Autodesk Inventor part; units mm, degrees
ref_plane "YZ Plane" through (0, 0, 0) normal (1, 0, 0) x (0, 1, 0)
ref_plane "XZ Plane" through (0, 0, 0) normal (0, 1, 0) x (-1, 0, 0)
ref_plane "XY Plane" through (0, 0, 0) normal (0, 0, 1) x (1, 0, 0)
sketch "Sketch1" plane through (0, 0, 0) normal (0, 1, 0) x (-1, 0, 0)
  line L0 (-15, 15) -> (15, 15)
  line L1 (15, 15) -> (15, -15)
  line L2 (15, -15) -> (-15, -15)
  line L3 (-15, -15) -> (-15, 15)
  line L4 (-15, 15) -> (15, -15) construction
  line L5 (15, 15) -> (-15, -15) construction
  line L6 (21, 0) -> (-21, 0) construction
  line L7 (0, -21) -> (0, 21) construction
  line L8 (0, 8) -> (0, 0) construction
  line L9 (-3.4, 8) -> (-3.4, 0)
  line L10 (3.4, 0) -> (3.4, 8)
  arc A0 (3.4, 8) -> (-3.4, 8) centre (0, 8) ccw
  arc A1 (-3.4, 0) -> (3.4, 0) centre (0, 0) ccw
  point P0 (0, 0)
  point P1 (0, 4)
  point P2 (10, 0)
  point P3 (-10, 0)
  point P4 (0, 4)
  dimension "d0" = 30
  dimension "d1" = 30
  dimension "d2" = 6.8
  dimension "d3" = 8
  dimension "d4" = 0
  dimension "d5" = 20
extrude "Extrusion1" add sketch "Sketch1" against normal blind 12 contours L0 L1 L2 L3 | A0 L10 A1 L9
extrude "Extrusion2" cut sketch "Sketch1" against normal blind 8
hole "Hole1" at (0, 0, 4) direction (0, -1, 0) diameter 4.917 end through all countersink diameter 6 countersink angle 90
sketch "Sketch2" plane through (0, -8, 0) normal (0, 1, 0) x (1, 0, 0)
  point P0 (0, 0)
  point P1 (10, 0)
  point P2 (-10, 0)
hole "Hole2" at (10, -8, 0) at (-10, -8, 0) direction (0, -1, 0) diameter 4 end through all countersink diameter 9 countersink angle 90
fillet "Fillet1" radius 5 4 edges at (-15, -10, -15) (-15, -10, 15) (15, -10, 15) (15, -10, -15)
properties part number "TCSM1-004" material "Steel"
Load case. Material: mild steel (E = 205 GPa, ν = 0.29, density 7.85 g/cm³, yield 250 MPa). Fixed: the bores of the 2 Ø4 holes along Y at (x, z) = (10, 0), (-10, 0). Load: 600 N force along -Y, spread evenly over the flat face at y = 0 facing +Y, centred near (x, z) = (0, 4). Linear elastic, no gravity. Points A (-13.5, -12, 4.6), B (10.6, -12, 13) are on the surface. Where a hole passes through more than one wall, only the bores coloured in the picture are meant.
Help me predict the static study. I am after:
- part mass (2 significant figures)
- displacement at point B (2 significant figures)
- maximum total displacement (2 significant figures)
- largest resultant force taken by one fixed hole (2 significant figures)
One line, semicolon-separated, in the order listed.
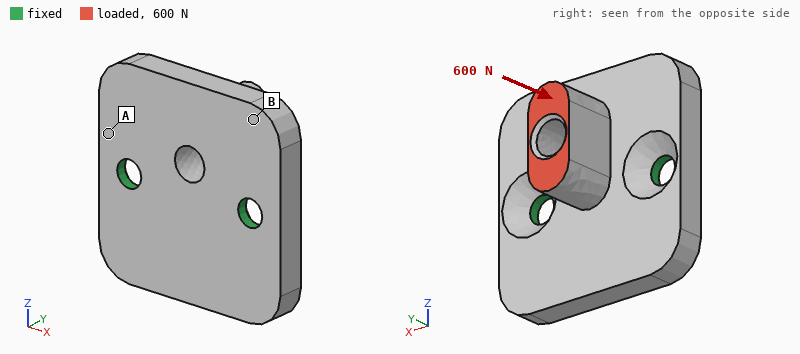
30 g; 8.3 µm; 12 µm; 380 N
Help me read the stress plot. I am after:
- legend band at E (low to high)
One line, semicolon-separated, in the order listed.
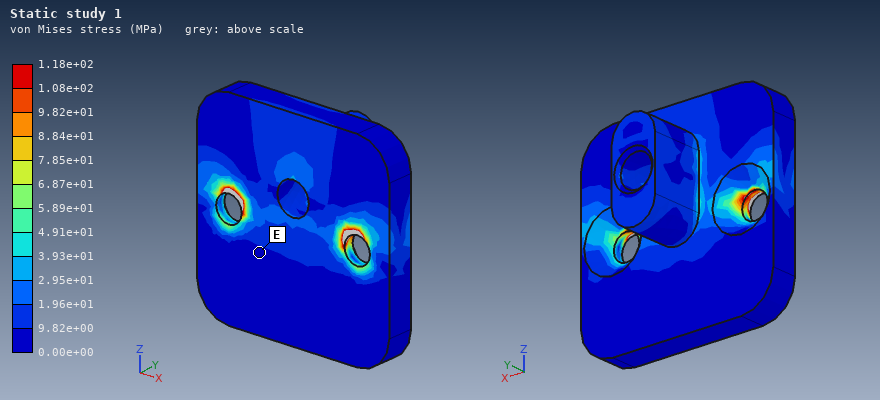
0.00e+00 to 9.82e+00 MPa
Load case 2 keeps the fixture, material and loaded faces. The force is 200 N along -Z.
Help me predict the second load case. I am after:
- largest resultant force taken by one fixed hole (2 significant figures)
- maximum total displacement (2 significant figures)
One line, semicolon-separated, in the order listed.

100 N; 9.9 µm
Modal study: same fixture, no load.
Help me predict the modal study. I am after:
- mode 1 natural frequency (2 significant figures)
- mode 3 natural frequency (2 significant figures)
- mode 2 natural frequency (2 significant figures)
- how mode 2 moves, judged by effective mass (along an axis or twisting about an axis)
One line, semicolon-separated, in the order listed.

7000 Hz; 18 kHz; 14 kHz; along Y
